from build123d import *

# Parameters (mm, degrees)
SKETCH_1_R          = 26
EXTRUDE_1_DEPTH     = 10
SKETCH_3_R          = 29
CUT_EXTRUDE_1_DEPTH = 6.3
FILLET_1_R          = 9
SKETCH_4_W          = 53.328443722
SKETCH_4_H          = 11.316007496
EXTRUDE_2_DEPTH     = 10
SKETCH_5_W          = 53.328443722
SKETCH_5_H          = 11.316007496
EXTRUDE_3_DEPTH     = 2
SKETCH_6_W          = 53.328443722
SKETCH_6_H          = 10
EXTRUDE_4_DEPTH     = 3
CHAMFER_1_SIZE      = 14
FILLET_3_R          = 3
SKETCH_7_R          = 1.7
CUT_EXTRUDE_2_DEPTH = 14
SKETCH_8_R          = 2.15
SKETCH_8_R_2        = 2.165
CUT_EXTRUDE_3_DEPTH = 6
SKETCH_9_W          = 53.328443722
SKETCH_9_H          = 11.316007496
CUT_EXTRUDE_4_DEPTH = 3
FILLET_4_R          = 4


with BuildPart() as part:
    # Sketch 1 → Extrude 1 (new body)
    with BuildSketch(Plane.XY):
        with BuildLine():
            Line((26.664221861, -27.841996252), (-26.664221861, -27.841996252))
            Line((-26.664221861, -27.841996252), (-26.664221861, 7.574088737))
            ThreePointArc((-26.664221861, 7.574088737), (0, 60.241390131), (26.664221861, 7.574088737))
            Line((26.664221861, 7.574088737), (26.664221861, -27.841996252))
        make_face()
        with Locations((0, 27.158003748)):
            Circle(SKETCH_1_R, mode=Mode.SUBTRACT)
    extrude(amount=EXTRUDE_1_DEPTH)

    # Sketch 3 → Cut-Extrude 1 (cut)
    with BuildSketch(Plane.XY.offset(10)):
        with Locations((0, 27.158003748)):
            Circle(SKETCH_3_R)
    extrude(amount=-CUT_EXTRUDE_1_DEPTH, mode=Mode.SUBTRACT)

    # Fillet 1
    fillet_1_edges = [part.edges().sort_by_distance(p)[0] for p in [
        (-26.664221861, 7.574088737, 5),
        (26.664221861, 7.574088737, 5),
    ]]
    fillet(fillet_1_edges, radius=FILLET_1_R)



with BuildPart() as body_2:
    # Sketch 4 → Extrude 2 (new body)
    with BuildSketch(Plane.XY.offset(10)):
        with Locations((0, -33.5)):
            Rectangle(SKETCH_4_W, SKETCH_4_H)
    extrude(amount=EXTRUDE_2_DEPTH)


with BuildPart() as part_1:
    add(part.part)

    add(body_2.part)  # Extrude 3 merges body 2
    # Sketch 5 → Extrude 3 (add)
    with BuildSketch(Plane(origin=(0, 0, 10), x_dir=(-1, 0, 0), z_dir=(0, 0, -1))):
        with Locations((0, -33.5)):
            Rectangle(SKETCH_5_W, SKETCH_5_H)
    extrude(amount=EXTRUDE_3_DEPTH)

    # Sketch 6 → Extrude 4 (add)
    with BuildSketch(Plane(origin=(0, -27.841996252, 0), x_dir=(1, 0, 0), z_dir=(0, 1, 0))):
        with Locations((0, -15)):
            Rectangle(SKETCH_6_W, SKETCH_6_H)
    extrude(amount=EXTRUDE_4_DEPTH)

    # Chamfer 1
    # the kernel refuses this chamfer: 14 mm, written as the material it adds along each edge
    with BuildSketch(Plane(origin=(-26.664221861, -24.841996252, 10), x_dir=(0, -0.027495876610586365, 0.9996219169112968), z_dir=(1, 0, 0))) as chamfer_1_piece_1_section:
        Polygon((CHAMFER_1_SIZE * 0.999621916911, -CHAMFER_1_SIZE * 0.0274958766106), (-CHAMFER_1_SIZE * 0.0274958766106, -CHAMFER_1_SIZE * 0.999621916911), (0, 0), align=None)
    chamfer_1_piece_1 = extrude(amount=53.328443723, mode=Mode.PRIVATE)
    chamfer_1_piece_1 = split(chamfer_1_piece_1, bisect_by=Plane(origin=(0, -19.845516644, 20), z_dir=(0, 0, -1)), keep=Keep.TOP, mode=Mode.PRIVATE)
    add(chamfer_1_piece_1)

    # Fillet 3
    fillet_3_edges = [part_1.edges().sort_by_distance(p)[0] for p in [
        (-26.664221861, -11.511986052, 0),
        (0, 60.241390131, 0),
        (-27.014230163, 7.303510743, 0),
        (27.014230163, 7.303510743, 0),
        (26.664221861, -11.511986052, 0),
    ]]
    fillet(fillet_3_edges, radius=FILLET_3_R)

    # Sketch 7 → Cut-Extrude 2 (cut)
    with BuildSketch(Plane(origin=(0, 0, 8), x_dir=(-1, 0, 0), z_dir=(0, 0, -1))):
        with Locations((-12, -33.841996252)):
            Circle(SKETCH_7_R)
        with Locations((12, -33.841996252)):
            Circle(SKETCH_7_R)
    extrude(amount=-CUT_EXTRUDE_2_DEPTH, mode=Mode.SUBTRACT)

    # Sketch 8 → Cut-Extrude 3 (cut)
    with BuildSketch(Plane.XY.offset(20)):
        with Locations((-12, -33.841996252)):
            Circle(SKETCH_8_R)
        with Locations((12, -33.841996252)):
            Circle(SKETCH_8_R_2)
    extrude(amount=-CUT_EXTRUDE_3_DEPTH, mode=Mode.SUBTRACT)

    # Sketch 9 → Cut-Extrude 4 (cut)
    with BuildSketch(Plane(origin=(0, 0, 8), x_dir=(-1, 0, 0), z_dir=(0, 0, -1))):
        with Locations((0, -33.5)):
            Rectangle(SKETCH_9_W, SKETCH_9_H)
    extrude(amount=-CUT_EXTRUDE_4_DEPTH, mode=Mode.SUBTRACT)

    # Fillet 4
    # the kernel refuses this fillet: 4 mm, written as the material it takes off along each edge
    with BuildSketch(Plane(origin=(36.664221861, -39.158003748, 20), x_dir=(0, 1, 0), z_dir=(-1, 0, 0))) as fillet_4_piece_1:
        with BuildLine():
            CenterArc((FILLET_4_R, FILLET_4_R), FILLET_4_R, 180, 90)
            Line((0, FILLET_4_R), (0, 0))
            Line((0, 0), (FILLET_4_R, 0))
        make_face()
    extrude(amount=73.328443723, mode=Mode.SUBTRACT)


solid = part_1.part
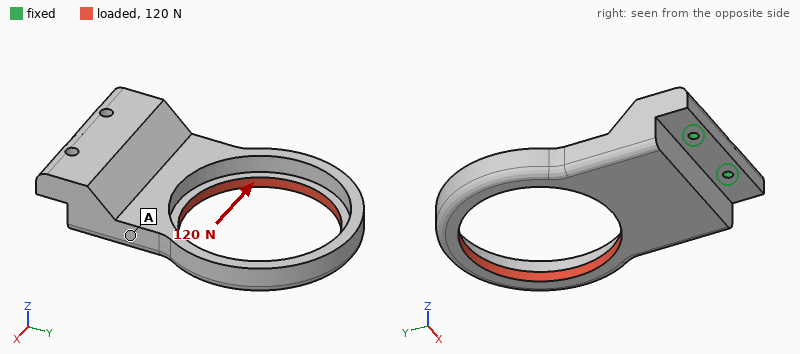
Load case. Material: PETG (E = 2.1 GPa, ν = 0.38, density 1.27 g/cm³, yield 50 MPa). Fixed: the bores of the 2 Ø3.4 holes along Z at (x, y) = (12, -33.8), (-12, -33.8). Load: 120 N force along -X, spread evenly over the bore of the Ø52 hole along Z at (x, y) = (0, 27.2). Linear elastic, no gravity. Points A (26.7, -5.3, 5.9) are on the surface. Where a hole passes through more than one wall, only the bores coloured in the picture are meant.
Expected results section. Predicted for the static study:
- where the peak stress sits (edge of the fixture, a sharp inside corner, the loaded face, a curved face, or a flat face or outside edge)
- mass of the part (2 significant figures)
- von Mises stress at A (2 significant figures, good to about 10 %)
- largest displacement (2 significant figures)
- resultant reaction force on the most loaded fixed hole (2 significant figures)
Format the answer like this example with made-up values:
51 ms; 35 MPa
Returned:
edge of the fixture; 44 g; 2.9 MPa; 1.4 mm; 300 N
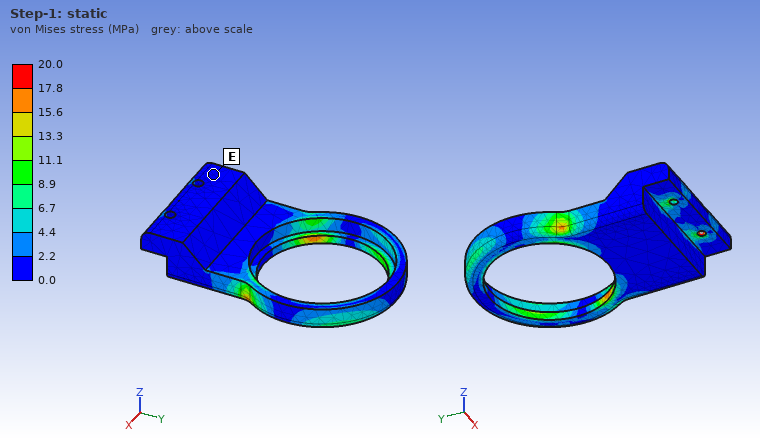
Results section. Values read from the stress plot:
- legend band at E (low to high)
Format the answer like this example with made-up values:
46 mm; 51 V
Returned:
0.0 to 2.2 MPa
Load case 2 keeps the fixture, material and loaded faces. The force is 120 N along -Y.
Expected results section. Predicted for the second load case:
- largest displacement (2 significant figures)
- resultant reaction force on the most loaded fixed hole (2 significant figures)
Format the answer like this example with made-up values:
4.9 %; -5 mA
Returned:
1.4 mm; 60 N
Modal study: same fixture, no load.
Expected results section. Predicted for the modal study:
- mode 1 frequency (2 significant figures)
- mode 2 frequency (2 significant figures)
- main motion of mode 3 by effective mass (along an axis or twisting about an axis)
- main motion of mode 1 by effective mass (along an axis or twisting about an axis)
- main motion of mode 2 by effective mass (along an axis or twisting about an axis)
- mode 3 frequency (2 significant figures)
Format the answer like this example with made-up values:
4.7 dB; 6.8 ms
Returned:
190 Hz; 440 Hz; along Z; along Z; along X; 670 Hz
